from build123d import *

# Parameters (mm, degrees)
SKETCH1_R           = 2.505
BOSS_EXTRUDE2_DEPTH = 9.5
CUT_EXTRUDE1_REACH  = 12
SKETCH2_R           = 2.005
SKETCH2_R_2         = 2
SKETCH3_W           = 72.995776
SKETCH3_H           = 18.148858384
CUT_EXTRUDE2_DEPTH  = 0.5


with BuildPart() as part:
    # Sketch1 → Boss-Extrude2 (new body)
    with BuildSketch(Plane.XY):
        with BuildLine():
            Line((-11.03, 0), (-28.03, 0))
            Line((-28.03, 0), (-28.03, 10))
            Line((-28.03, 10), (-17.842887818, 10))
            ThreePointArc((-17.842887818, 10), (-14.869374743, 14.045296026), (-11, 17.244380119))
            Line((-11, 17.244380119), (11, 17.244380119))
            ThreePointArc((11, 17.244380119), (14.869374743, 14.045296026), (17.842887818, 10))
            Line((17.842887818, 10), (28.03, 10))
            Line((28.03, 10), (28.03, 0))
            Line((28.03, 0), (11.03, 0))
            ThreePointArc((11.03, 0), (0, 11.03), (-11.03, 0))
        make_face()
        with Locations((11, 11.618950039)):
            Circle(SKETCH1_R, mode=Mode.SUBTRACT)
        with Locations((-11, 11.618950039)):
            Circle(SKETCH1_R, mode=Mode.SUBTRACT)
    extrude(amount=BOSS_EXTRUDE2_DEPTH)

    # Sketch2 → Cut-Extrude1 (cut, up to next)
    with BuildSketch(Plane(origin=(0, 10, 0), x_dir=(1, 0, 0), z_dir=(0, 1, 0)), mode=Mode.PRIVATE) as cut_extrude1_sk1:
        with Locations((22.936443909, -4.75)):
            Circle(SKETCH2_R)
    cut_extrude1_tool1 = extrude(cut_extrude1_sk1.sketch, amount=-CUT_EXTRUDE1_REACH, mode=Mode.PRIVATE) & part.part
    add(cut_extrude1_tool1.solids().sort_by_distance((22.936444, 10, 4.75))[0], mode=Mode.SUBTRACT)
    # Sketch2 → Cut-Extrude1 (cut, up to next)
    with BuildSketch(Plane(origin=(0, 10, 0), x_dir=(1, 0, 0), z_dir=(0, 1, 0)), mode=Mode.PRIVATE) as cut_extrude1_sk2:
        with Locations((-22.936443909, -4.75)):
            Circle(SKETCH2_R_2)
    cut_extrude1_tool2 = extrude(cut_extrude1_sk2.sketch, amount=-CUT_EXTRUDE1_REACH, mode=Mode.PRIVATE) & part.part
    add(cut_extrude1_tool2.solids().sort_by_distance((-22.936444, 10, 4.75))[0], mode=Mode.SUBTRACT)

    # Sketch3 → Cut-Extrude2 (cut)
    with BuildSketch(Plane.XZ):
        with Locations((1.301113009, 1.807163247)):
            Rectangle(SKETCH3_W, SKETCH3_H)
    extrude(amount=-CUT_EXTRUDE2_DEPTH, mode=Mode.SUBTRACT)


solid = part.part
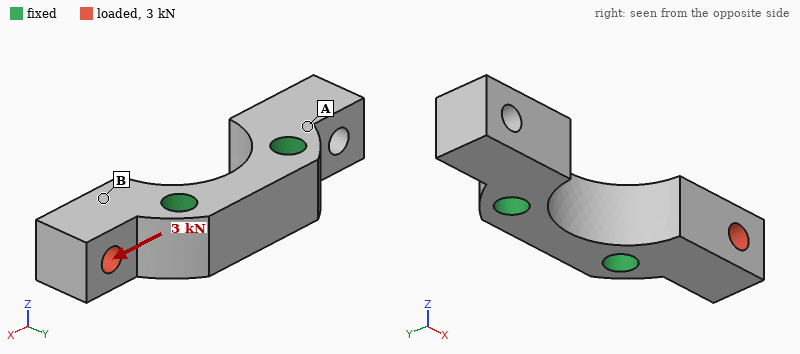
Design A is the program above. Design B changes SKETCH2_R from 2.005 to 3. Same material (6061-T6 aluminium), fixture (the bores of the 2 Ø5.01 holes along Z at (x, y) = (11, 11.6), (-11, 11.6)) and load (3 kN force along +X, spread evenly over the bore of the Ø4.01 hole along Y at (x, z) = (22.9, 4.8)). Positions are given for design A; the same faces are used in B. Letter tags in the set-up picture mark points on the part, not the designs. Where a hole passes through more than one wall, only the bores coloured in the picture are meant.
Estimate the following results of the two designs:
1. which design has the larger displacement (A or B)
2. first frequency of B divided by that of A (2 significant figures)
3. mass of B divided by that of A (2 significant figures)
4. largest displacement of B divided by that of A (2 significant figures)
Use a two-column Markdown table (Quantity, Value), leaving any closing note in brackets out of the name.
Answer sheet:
| Quantity | Value |
|---|---|
| which design has the larger displacement | B |
| first frequency of B divided by that of A | 1.0 |
| mass of B divided by that of A | 0.97 |
| largest displacement of B divided by that of A | 1.1 |
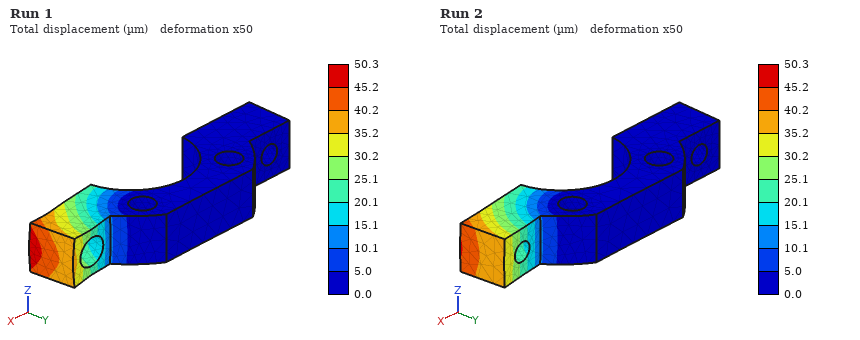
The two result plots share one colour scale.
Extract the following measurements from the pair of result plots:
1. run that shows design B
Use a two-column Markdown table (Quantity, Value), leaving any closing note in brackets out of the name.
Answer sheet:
| Quantity | Value |
|---|---|
| run that shows design B | Run 1 |
